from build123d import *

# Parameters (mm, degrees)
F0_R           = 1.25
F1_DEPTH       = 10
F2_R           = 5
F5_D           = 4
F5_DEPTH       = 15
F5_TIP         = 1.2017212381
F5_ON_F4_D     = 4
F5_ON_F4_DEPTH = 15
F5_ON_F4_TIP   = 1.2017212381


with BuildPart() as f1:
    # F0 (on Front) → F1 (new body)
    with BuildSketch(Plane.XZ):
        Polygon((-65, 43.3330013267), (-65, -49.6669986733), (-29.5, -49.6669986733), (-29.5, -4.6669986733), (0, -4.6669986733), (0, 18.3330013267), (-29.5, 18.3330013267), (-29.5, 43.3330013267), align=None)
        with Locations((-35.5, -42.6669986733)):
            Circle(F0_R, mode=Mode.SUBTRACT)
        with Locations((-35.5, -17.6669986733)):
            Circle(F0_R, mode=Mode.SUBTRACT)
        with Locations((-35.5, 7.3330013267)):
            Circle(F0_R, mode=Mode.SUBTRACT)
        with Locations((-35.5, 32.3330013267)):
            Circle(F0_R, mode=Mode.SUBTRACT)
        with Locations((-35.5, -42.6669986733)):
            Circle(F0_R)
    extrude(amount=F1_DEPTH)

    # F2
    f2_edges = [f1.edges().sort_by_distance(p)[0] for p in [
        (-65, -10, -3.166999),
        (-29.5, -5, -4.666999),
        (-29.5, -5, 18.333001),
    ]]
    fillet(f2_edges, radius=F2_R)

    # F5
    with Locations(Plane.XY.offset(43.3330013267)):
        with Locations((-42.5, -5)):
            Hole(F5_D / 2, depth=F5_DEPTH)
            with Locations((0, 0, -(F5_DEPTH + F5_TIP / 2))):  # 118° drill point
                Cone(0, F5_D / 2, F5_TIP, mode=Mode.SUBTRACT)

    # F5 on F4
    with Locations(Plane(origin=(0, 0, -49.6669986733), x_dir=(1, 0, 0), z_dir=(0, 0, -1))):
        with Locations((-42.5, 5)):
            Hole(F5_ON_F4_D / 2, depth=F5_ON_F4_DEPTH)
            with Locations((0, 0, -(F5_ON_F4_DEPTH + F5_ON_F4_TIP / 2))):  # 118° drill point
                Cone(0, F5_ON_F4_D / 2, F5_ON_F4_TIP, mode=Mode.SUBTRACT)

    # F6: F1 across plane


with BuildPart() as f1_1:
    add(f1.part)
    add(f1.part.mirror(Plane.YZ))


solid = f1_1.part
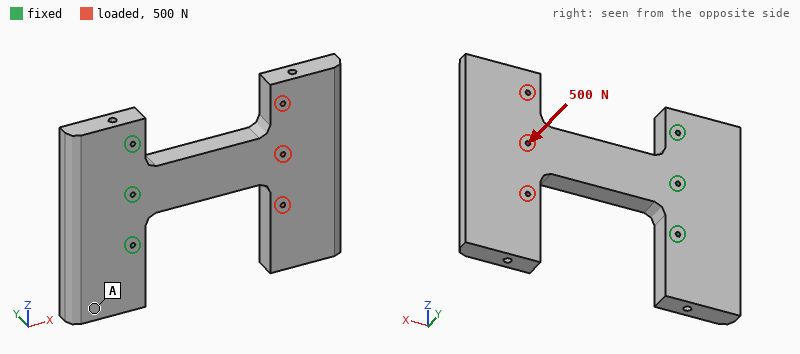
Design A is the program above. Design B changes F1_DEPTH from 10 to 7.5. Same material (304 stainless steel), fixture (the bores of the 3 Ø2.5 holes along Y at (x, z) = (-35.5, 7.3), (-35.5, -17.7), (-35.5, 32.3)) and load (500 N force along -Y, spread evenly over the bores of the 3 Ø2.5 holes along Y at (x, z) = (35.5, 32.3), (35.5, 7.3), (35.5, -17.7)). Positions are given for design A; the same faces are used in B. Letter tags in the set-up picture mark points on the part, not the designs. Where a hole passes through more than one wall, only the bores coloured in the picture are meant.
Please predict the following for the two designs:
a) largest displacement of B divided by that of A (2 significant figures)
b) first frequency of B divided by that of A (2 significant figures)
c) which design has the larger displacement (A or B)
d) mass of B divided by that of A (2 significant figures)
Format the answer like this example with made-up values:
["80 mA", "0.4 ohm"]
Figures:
["2.3", "0.76", "B", "0.74"]
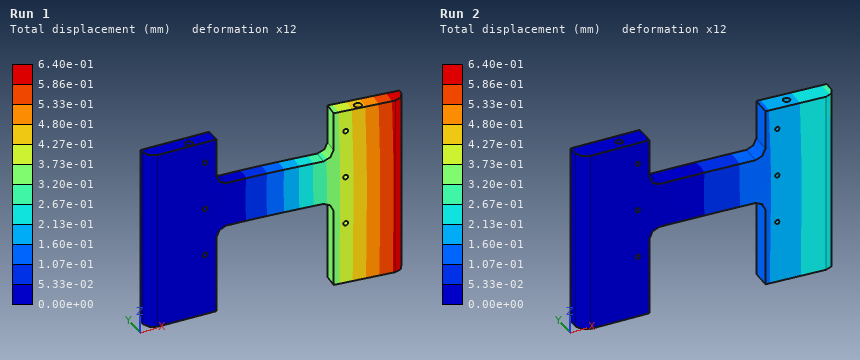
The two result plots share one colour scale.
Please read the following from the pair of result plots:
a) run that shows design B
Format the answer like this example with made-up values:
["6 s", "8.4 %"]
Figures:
["Run 1"]
